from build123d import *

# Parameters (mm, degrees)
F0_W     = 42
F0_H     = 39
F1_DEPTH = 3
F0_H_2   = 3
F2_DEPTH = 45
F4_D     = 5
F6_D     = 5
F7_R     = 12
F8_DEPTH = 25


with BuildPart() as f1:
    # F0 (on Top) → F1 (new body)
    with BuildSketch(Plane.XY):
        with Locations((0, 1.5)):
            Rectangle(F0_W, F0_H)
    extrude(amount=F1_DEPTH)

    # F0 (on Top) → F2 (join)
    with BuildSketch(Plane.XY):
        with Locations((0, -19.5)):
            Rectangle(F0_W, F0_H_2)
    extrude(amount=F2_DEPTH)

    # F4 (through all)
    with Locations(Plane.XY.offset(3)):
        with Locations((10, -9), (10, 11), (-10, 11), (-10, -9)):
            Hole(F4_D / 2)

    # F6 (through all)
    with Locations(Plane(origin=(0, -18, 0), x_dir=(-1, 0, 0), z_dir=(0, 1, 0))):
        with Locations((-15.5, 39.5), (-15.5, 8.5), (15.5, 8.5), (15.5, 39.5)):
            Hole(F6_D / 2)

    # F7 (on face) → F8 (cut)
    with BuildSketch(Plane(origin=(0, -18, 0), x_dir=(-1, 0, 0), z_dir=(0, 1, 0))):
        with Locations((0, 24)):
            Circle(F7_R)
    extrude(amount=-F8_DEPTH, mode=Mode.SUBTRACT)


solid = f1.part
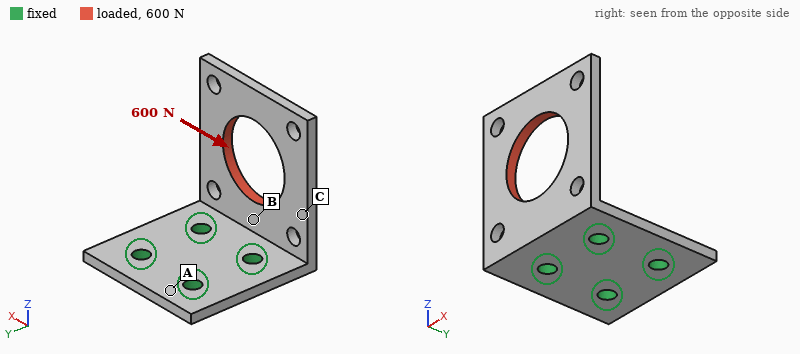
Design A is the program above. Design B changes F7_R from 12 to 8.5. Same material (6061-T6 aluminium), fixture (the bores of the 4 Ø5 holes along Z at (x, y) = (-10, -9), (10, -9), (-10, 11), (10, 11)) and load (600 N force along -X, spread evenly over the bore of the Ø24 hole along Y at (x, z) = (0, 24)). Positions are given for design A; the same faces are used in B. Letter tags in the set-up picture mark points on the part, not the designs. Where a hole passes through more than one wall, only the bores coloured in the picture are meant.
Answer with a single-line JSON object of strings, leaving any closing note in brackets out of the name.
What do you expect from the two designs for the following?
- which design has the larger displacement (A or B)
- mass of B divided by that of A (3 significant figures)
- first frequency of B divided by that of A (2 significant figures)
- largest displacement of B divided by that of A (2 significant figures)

{"which design has the larger displacement": "A", "mass of B divided by that of A": "1.08", "first frequency of B divided by that of A": "1.0", "largest displacement of B divided by that of A": "0.90"}
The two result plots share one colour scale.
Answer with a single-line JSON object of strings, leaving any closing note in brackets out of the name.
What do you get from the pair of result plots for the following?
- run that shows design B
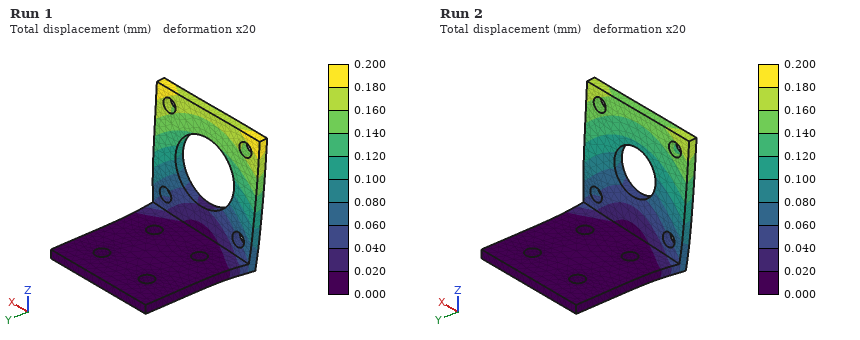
{"run that shows design B": "Run 2"}
